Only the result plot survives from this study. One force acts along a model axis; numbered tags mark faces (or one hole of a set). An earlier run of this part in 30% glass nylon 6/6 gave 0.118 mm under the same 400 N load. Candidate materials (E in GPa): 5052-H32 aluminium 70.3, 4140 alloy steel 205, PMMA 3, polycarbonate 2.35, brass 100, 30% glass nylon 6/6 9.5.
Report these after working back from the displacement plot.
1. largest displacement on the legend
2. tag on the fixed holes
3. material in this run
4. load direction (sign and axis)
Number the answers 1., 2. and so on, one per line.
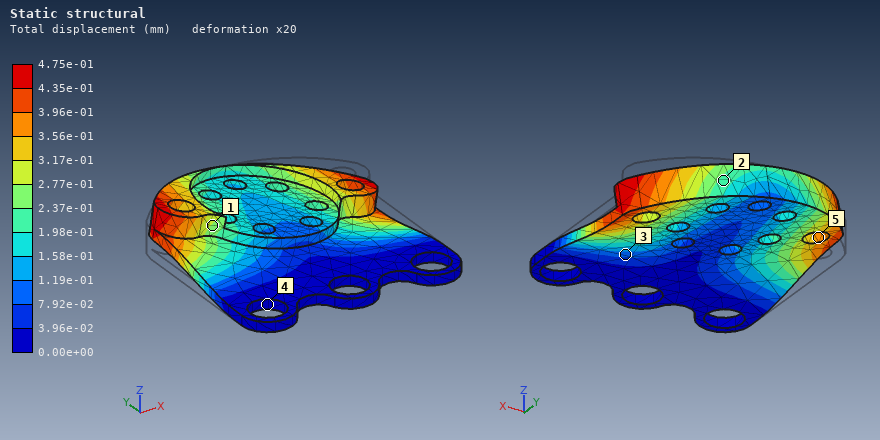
1. 4.75e-01 mm
2. 4
3. polycarbonate
4. +X
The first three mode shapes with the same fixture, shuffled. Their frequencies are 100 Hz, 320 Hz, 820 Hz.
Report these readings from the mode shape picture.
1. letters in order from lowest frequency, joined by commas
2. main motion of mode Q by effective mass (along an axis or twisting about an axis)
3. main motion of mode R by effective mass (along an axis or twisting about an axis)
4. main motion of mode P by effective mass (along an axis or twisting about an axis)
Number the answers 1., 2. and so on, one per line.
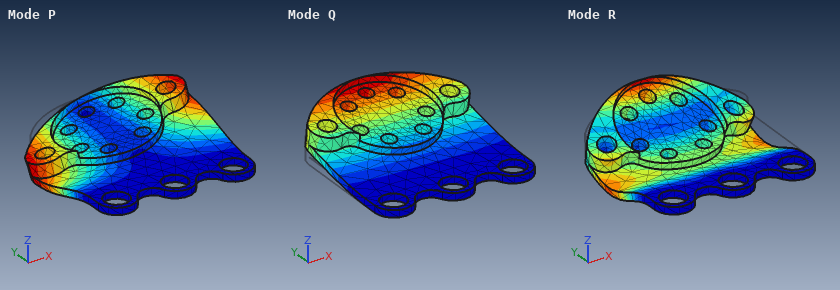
1. Q, P, R
2. along Z
3. along Z
4. twisting about Y
